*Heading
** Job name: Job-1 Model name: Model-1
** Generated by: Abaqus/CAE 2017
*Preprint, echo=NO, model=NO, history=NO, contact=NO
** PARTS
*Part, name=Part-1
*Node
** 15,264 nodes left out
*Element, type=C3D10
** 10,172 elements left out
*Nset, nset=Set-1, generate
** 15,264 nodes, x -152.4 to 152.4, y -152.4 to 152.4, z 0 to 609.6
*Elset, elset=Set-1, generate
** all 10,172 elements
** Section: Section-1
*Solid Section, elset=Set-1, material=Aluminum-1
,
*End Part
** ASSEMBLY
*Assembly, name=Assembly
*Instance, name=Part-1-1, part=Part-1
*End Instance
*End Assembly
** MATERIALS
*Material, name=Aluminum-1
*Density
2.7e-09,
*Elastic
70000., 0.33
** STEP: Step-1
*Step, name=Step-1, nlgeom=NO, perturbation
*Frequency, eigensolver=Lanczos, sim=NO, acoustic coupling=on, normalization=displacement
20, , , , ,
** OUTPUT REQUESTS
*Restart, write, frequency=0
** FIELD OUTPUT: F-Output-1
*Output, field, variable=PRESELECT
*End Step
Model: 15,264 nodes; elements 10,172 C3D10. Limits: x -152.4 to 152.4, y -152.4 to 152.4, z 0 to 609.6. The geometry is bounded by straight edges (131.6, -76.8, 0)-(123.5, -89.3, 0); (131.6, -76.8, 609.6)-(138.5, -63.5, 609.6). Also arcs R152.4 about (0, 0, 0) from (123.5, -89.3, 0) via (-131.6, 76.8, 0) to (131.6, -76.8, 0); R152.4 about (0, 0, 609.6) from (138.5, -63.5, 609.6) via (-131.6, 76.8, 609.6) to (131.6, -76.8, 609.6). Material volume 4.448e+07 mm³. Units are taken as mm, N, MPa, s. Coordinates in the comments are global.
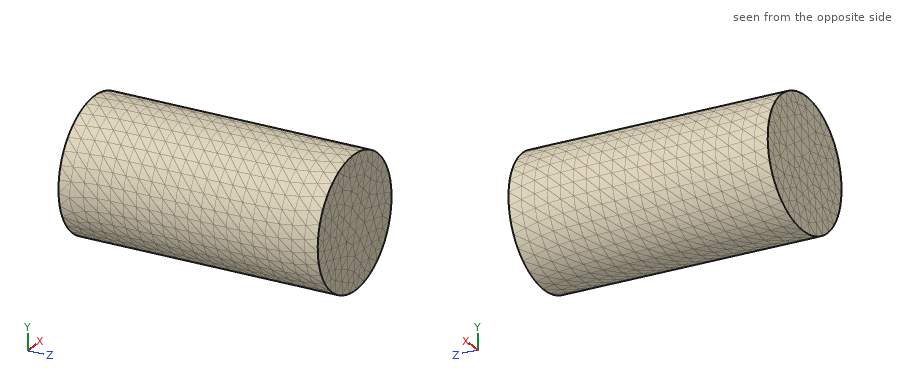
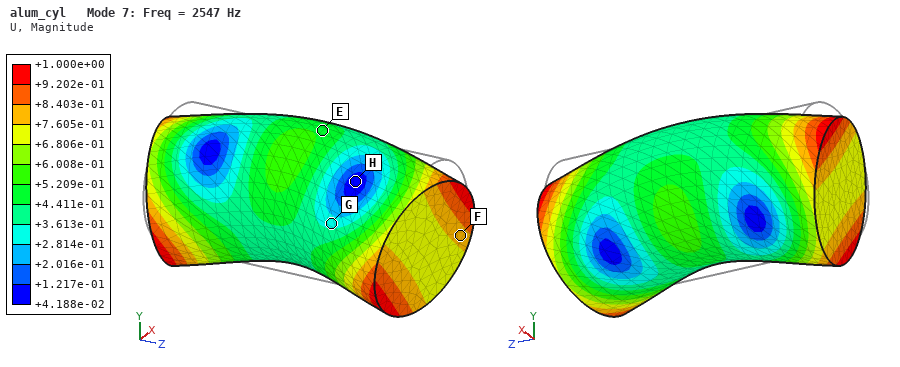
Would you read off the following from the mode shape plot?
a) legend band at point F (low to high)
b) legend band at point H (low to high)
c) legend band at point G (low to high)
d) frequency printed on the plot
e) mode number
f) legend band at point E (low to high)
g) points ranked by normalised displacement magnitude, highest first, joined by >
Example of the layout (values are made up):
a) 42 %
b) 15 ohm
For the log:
a) +7.605e-01 to +8.403e-01
b) +4.188e-02 to +1.217e-01
c) +2.814e-01 to +3.613e-01
d) 2547 Hz
e) 7
f) +4.411e-01 to +5.209e-01
g) F > E > G > H
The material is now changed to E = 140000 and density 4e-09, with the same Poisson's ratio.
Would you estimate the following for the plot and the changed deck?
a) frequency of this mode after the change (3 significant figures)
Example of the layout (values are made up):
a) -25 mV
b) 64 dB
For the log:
a) 2960 Hz
